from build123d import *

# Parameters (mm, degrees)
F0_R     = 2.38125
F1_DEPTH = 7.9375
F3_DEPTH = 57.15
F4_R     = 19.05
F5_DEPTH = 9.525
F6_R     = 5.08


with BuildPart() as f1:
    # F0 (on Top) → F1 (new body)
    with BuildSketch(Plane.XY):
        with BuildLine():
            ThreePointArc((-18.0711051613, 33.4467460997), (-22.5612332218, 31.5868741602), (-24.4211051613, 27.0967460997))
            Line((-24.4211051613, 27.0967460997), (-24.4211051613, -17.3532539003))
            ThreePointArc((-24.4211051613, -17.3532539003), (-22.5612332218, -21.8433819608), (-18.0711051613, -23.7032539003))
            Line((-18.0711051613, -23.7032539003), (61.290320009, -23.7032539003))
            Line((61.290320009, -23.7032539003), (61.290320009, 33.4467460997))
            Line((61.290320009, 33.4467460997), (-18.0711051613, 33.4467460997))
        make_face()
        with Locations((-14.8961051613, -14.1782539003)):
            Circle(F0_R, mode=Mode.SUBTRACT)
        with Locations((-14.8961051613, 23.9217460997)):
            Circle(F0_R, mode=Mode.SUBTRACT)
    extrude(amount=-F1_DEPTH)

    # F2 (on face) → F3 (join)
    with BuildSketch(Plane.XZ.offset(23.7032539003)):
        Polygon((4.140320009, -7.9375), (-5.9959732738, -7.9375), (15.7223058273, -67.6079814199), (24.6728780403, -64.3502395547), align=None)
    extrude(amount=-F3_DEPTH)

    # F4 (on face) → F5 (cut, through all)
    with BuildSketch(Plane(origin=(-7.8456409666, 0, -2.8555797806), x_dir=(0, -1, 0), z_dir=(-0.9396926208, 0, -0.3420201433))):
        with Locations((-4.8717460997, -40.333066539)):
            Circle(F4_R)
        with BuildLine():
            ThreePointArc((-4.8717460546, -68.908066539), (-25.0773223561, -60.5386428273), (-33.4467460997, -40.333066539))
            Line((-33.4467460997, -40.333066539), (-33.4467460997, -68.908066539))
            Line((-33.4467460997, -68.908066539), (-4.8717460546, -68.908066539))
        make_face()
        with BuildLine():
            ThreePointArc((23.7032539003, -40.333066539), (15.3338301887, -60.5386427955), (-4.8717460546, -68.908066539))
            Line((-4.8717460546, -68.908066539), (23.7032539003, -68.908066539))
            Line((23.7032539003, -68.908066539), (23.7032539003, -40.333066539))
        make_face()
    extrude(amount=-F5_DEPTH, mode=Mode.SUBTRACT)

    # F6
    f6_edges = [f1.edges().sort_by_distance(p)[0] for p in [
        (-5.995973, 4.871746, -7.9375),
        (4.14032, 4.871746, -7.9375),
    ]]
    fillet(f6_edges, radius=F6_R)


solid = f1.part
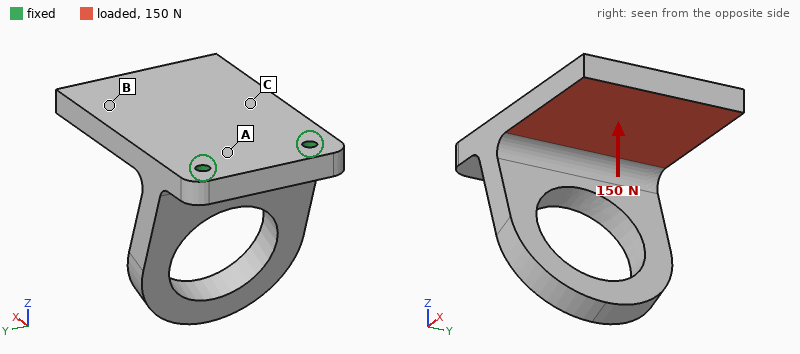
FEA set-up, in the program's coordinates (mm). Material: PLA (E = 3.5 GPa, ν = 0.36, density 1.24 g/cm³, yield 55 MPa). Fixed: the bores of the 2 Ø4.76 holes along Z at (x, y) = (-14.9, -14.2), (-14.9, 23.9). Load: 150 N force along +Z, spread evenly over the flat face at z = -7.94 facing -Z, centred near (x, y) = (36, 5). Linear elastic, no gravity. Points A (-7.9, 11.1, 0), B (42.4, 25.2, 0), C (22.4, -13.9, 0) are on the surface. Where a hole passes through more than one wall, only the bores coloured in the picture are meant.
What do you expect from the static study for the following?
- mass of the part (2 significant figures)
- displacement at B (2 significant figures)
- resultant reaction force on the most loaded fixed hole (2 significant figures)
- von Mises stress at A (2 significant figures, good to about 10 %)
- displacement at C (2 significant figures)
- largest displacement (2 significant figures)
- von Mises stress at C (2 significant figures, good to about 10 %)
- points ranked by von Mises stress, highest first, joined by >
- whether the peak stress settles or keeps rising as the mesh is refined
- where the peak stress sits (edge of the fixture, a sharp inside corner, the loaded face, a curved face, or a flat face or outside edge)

73 g
0.84 mm
76 N
6.6 MPa
0.45 mm
1.2 mm
3.6 MPa
A > C > B
keeps rising
edge of the fixture
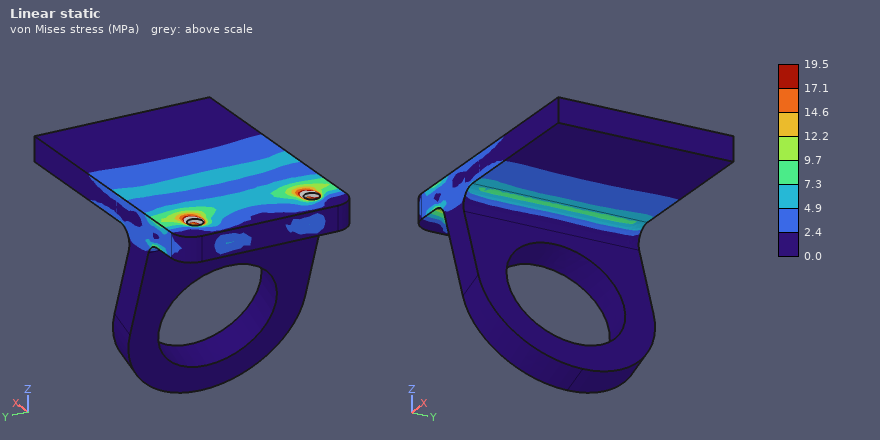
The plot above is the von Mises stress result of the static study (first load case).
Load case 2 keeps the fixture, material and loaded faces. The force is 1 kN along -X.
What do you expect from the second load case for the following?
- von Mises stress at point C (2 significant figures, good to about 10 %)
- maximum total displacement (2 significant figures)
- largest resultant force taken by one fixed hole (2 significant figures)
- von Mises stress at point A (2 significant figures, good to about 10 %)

3.2 MPa
0.94 mm
500 N
2.8 MPa
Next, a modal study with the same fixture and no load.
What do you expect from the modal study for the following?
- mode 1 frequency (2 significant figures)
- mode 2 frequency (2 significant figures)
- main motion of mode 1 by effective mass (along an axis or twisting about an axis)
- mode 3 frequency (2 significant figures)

350 Hz
760 Hz
along Z
1100 Hz
